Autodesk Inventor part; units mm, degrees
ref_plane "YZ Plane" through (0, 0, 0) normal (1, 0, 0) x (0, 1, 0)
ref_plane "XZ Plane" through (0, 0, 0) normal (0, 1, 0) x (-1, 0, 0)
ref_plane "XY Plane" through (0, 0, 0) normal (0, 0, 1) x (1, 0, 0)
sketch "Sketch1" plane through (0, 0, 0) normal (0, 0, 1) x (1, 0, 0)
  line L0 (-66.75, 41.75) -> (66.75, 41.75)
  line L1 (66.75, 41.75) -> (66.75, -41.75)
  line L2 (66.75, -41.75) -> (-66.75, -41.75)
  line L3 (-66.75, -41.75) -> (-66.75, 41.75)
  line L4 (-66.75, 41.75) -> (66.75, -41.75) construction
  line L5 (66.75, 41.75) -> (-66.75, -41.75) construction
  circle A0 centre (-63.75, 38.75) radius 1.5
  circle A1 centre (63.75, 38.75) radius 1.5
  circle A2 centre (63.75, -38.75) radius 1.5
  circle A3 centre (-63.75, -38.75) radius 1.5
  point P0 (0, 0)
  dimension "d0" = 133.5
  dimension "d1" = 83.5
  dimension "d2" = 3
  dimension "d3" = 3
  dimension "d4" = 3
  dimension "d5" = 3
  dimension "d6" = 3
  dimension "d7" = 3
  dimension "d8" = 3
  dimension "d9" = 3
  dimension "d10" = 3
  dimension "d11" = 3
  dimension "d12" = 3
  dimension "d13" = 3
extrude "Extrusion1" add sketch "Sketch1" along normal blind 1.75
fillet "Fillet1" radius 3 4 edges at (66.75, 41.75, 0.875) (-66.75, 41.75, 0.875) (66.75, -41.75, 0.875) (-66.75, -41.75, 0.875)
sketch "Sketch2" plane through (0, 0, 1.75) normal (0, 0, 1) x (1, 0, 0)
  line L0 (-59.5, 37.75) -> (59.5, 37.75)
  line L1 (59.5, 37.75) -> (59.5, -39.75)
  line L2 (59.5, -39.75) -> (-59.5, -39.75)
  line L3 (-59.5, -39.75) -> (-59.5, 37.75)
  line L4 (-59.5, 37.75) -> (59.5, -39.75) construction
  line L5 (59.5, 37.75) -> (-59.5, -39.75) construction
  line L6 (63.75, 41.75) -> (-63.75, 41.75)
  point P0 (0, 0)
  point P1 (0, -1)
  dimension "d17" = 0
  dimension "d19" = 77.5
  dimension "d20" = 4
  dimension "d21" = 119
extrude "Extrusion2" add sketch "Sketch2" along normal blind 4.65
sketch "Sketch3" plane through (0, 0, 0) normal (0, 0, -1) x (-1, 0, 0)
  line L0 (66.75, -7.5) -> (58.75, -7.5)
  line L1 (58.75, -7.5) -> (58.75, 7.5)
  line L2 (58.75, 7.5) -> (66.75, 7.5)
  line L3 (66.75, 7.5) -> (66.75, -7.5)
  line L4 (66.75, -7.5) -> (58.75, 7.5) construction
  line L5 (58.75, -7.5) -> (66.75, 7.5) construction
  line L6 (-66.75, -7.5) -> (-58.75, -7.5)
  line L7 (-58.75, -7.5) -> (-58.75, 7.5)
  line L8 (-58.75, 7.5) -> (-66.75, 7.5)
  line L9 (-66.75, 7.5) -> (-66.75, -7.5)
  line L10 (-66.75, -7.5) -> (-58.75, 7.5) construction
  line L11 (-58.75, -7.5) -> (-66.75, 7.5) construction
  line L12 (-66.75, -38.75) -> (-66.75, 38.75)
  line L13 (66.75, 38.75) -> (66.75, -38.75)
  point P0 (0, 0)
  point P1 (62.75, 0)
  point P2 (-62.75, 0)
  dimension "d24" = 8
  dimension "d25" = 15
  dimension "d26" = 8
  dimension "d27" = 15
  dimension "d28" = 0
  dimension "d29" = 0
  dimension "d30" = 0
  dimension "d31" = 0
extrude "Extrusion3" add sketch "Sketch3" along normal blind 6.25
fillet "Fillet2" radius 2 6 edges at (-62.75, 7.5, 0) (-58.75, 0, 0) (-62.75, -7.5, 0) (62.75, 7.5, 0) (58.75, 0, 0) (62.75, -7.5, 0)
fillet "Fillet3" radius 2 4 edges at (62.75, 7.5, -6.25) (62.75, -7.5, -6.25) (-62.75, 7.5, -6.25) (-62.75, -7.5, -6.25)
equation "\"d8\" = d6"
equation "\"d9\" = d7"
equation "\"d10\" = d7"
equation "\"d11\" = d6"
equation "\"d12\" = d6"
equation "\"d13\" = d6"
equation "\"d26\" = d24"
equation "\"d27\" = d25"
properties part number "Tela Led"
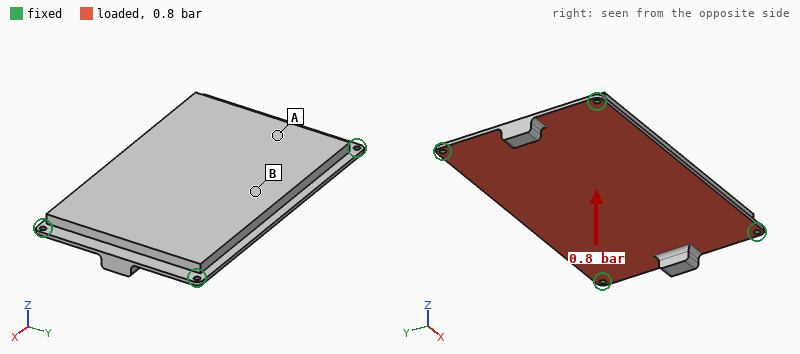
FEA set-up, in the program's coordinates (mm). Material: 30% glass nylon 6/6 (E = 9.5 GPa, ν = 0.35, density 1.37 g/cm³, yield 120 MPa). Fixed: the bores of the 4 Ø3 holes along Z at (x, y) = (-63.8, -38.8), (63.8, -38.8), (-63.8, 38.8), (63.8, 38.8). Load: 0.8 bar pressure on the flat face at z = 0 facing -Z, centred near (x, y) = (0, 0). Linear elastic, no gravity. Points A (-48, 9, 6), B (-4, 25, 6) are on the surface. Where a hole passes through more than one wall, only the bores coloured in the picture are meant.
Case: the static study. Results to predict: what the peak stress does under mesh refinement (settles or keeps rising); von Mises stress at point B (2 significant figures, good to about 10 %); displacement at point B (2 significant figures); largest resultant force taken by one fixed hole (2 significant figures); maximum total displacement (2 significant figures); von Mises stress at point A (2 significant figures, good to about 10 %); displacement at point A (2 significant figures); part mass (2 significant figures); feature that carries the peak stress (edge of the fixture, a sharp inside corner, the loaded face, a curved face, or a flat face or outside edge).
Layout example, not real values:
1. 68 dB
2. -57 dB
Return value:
1. keeps rising
2. 19 MPa
3. 0.96 mm
4. 670 N
5. 1.0 mm
6. 7.7 MPa
7. 0.45 mm
8. 87 g
9. edge of the fixture
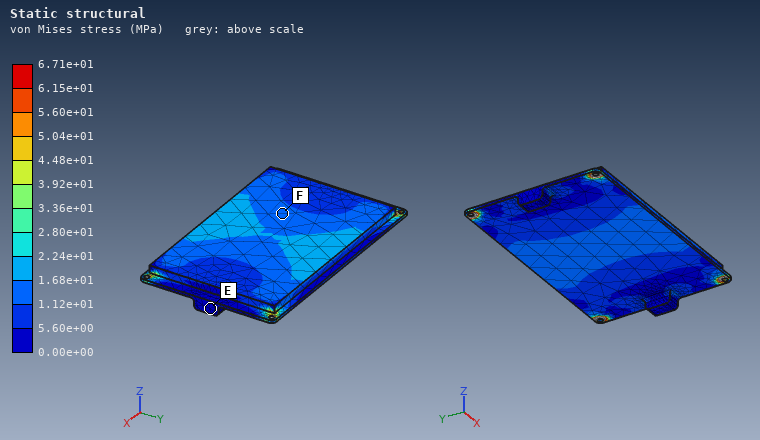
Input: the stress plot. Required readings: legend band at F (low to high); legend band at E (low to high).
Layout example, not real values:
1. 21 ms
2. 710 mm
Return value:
1. 1.12e+01 to 1.68e+01 MPa
2. 0.00e+00 to 5.60e+00 MPa
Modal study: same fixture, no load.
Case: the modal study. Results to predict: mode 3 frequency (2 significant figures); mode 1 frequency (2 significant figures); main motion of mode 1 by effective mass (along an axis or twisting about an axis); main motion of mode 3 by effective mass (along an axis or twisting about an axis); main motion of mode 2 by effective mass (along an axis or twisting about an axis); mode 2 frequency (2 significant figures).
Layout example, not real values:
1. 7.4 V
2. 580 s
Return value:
1. 1400 Hz
2. 570 Hz
3. along Z
4. twisting about Y
5. twisting about X
6. 1100 Hz
